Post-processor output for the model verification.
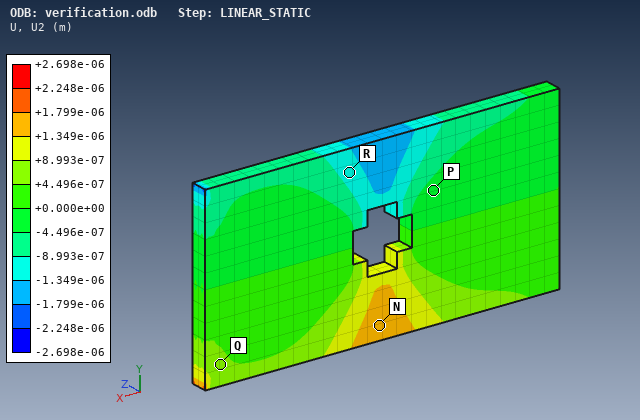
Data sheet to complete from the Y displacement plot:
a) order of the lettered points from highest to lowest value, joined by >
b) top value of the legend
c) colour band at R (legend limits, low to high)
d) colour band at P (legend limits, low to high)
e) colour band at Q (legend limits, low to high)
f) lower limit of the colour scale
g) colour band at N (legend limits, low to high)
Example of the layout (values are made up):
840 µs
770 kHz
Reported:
N > Q > P > R
+2.698e-06 m
-1.349e-06 to -8.993e-07 m
-4.496e-07 to +0.000e+00 m
+4.496e-07 to +8.993e-07 m
-2.698e-06 m
+1.349e-06 to +1.799e-06 m
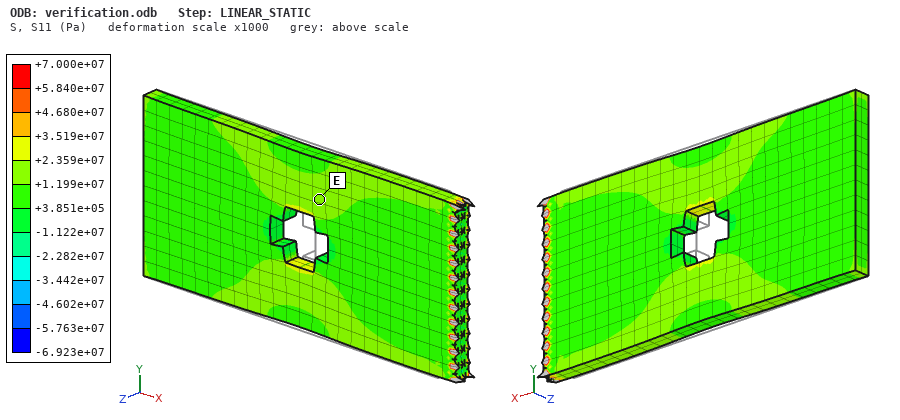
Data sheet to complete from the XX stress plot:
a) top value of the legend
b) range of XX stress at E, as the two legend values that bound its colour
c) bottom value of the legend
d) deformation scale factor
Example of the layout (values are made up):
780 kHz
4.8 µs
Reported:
+7.000e+07 Pa
+1.199e+07 to +2.359e+07 Pa
-6.923e+07 Pa
1000
